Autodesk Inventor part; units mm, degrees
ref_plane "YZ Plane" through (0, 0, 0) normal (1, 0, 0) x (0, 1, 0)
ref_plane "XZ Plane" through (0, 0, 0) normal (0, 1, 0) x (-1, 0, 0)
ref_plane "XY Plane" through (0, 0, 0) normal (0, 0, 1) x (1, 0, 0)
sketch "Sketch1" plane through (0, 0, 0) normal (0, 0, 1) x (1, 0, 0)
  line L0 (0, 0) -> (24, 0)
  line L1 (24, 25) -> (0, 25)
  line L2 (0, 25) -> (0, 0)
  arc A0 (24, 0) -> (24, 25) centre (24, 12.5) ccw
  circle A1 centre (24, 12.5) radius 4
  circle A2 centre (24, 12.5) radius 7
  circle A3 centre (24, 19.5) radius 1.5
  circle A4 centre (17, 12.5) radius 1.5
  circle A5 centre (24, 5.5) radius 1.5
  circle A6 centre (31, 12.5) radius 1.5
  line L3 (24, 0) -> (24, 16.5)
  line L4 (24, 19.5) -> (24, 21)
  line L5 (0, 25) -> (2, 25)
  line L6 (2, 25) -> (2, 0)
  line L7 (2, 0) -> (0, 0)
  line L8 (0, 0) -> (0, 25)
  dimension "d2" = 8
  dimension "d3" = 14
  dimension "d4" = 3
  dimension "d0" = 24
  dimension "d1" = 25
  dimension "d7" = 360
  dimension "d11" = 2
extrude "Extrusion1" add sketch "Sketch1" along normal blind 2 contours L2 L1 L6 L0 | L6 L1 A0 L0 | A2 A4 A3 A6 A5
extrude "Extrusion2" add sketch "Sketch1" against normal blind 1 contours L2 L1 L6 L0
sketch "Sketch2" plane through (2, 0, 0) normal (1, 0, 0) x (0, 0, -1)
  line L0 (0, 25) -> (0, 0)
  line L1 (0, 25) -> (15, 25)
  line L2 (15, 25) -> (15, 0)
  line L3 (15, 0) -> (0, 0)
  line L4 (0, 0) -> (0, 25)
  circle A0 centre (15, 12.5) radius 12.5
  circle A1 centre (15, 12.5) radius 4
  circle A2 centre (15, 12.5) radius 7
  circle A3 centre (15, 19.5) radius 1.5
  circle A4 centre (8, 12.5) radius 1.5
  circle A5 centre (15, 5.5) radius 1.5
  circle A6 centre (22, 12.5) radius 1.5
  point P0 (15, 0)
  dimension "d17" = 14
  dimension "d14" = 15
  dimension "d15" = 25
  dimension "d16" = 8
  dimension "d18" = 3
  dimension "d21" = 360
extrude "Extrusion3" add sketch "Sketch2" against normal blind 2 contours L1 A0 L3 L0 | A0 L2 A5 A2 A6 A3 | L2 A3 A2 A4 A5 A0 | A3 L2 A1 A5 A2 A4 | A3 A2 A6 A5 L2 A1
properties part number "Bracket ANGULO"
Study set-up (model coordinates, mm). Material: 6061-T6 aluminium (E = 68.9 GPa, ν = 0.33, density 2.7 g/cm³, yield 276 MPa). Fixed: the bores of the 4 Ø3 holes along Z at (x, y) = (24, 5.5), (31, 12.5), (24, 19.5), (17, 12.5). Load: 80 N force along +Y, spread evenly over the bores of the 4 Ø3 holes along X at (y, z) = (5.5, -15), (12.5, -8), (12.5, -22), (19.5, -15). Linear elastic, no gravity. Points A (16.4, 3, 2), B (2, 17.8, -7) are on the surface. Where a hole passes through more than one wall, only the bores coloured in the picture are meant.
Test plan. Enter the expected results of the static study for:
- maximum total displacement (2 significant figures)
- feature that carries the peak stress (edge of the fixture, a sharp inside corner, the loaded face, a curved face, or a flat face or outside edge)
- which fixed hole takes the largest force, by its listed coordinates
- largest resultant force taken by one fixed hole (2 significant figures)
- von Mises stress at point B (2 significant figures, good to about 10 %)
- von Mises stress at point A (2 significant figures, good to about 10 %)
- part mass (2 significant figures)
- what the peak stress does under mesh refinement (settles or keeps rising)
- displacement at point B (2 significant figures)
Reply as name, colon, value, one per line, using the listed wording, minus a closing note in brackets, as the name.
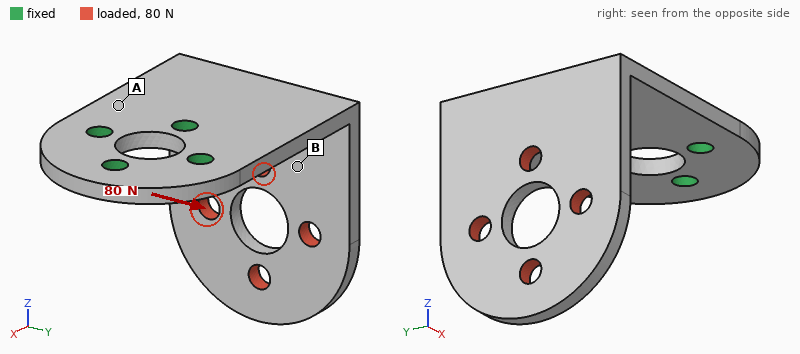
maximum total displacement: 0.28 mm
feature that carries the peak stress: edge of the fixture
which fixed hole takes the largest force, by its listed coordinates: (17, 12.5)
largest resultant force taken by one fixed hole: 94 N
von Mises stress at point B: 14 MPa
von Mises stress at point A: 46 MPa
part mass: 7.1 g
what the peak stress does under mesh refinement: keeps rising
displacement at point B: 0.094 mm
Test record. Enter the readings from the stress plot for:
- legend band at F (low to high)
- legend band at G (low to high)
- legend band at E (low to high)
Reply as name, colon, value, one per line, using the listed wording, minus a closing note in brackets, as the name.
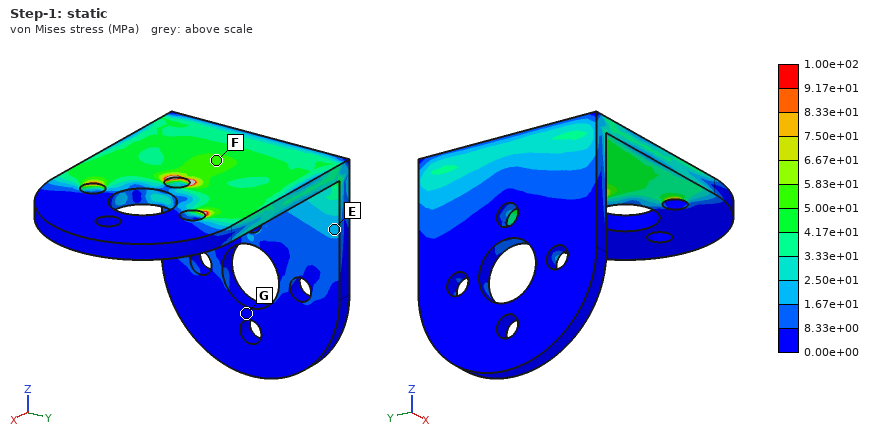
legend band at F: 5.00e+01 to 5.83e+01 MPa
legend band at G: 0.00e+00 to 8.33e+00 MPa
legend band at E: 1.67e+01 to 2.50e+01 MPa
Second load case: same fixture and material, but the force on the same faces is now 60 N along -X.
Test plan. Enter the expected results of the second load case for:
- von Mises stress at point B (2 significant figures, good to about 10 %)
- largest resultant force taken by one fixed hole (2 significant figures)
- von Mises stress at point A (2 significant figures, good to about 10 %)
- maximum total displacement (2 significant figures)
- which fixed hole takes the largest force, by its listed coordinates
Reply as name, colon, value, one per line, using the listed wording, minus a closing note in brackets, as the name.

von Mises stress at point B: 29 MPa
largest resultant force taken by one fixed hole: 79 N
von Mises stress at point A: 32 MPa
maximum total displacement: 0.53 mm
which fixed hole takes the largest force, by its listed coordinates: (17, 12.5)
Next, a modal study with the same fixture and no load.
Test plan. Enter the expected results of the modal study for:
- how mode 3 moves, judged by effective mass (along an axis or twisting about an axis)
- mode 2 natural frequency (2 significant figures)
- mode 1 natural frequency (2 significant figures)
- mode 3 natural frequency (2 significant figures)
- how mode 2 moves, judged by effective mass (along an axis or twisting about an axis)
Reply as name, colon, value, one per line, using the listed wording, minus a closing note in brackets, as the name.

how mode 3 moves, judged by effective mass: along Z
mode 2 natural frequency: 1900 Hz
mode 1 natural frequency: 1300 Hz
mode 3 natural frequency: 3600 Hz
how mode 2 moves, judged by effective mass: along Y
